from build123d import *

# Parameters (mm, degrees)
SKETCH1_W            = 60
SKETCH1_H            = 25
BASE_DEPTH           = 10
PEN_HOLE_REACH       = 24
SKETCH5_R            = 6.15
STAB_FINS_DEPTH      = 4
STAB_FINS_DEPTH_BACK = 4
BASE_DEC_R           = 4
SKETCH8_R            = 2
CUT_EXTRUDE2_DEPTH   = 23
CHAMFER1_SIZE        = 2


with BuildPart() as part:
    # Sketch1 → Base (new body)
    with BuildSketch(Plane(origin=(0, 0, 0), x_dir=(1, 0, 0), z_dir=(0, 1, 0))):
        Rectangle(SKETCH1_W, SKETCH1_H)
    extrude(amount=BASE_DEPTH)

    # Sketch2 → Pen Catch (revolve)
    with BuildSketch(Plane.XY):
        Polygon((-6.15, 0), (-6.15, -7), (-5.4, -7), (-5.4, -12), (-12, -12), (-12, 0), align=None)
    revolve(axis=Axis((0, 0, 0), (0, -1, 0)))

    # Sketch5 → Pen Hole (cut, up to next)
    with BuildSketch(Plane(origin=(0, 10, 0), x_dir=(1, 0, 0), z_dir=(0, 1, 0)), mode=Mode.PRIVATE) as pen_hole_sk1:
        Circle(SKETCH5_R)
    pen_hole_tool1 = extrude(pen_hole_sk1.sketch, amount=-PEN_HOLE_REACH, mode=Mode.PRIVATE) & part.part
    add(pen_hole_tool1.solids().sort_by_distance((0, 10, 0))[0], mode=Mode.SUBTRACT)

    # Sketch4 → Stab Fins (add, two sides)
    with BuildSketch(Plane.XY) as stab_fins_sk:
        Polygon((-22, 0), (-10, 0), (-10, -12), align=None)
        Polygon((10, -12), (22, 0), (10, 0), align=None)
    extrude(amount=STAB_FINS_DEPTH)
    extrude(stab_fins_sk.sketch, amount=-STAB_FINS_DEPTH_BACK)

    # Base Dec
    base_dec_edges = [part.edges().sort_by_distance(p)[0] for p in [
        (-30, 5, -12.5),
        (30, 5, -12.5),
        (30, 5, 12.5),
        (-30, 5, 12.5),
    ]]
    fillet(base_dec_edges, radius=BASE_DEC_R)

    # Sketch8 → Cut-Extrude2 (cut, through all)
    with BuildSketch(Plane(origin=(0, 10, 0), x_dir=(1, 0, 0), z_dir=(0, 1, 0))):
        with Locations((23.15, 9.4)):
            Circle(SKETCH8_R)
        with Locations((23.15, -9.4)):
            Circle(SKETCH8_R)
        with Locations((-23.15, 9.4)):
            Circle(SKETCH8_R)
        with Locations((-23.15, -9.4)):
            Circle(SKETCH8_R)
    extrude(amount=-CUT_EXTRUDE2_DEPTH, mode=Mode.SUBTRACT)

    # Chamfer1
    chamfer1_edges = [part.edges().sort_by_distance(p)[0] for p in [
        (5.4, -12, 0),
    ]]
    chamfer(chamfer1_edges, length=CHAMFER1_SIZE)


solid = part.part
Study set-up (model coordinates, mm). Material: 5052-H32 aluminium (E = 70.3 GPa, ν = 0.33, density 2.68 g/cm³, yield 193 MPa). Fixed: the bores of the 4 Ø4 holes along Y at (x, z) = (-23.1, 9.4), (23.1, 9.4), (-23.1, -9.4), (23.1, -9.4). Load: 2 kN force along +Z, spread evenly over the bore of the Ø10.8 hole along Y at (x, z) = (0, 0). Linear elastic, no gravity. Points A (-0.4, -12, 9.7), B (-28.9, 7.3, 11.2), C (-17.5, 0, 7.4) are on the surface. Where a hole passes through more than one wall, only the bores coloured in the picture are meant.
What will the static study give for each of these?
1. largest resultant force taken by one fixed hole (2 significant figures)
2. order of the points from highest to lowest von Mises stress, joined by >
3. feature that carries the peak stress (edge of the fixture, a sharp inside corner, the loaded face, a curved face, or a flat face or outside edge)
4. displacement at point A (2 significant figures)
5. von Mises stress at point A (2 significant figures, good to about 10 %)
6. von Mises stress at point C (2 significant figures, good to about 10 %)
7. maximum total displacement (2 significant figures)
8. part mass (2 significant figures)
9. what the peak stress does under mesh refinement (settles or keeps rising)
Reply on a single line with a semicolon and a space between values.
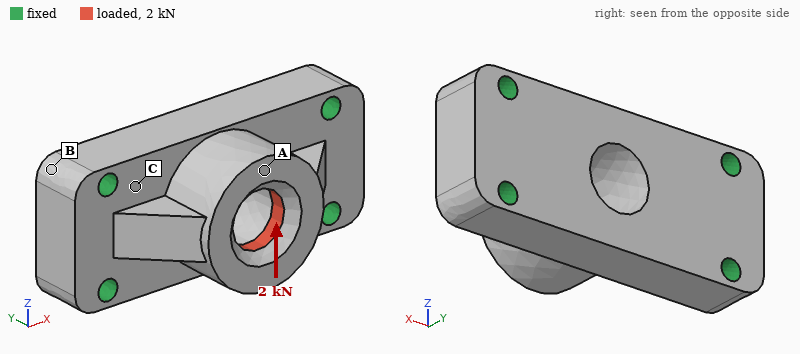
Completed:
980 N; C > A > B; edge of the fixture; 19 µm; 13 MPa; 22 MPa; 20 µm; 48 g; keeps rising
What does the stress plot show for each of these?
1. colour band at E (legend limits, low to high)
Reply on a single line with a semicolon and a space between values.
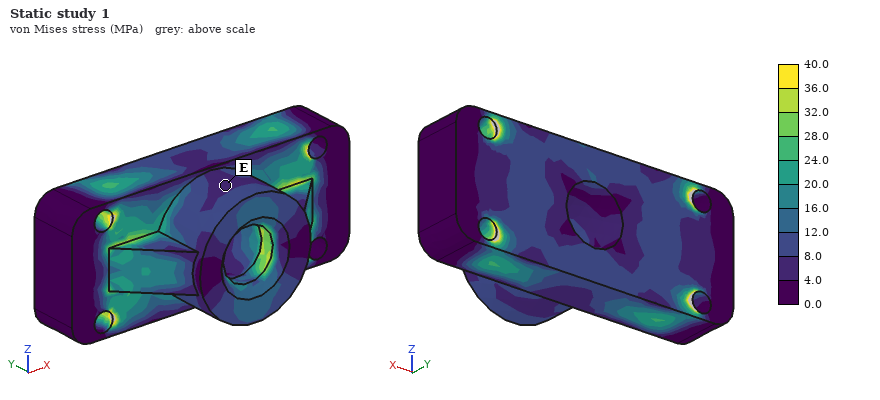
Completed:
4.0 to 8.0 MPa
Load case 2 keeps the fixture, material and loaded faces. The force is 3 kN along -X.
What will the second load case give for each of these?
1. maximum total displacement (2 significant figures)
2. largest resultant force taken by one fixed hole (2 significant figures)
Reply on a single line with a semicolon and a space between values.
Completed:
7.5 µm; 910 N
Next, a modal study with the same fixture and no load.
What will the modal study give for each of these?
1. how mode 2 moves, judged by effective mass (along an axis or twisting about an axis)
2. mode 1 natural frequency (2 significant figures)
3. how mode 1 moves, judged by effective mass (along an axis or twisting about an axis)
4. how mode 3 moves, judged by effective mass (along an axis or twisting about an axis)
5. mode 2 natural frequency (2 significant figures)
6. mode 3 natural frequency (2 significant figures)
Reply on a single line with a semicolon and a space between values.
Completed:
along Y; 17 kHz; along Z; along Z; 19 kHz; 29 kHz
